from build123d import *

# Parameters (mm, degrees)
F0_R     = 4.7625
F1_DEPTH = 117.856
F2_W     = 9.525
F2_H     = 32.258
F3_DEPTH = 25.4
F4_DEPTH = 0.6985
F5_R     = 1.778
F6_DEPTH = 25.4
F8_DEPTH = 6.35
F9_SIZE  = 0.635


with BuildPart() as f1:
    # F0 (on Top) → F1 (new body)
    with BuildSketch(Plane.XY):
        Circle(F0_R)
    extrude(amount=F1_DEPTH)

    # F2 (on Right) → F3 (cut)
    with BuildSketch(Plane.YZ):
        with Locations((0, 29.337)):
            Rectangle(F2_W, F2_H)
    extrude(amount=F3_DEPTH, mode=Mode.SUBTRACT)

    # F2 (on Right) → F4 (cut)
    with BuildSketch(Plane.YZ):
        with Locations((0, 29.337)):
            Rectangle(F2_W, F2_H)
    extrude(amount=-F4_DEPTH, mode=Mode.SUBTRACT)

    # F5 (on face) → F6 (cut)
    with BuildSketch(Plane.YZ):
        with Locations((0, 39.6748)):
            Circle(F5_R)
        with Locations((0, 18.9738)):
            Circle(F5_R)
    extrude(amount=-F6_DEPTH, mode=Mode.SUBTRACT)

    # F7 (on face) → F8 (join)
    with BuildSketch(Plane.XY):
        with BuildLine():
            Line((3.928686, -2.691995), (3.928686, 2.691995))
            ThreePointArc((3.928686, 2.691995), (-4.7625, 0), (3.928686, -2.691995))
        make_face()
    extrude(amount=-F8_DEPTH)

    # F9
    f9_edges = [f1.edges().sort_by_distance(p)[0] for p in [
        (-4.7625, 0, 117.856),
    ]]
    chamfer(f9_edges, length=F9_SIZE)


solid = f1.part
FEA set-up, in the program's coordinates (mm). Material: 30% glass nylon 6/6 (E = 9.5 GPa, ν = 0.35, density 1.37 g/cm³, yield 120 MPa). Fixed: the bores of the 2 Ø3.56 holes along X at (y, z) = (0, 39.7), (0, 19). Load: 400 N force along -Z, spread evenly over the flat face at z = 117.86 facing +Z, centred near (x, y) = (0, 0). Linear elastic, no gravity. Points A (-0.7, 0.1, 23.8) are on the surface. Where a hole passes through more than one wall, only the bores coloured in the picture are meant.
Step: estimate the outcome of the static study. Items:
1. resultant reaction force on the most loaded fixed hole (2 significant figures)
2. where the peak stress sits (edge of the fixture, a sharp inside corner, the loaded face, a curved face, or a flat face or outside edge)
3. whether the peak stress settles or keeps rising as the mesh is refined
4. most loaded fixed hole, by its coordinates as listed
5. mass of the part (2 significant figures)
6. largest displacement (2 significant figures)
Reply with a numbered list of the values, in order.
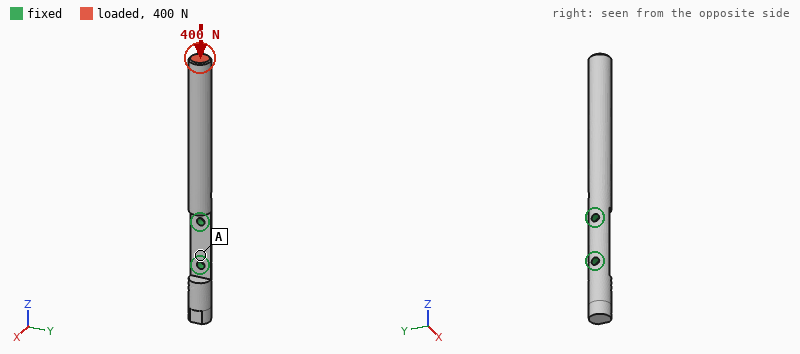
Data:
1. 380 N
2. edge of the fixture
3. keeps rising
4. (0, 39.7)
5. 10 g
6. 1.4 mm
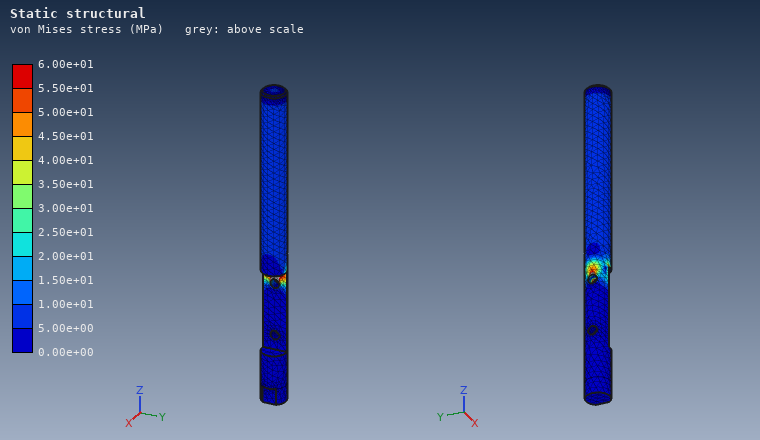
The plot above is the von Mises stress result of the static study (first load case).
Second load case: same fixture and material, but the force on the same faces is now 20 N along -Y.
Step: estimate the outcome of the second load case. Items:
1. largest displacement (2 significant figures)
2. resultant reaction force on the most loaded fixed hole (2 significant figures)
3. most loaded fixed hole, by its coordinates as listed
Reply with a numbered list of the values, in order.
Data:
1. 1.3 mm
2. 39 N
3. (0, 39.7)
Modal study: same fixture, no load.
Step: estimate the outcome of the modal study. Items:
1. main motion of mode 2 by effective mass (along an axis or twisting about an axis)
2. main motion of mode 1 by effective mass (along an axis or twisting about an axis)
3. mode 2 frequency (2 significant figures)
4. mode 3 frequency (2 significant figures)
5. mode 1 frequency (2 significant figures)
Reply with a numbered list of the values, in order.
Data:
1. along Y
2. along X
3. 430 Hz
4. 2000 Hz
5. 290 Hz
